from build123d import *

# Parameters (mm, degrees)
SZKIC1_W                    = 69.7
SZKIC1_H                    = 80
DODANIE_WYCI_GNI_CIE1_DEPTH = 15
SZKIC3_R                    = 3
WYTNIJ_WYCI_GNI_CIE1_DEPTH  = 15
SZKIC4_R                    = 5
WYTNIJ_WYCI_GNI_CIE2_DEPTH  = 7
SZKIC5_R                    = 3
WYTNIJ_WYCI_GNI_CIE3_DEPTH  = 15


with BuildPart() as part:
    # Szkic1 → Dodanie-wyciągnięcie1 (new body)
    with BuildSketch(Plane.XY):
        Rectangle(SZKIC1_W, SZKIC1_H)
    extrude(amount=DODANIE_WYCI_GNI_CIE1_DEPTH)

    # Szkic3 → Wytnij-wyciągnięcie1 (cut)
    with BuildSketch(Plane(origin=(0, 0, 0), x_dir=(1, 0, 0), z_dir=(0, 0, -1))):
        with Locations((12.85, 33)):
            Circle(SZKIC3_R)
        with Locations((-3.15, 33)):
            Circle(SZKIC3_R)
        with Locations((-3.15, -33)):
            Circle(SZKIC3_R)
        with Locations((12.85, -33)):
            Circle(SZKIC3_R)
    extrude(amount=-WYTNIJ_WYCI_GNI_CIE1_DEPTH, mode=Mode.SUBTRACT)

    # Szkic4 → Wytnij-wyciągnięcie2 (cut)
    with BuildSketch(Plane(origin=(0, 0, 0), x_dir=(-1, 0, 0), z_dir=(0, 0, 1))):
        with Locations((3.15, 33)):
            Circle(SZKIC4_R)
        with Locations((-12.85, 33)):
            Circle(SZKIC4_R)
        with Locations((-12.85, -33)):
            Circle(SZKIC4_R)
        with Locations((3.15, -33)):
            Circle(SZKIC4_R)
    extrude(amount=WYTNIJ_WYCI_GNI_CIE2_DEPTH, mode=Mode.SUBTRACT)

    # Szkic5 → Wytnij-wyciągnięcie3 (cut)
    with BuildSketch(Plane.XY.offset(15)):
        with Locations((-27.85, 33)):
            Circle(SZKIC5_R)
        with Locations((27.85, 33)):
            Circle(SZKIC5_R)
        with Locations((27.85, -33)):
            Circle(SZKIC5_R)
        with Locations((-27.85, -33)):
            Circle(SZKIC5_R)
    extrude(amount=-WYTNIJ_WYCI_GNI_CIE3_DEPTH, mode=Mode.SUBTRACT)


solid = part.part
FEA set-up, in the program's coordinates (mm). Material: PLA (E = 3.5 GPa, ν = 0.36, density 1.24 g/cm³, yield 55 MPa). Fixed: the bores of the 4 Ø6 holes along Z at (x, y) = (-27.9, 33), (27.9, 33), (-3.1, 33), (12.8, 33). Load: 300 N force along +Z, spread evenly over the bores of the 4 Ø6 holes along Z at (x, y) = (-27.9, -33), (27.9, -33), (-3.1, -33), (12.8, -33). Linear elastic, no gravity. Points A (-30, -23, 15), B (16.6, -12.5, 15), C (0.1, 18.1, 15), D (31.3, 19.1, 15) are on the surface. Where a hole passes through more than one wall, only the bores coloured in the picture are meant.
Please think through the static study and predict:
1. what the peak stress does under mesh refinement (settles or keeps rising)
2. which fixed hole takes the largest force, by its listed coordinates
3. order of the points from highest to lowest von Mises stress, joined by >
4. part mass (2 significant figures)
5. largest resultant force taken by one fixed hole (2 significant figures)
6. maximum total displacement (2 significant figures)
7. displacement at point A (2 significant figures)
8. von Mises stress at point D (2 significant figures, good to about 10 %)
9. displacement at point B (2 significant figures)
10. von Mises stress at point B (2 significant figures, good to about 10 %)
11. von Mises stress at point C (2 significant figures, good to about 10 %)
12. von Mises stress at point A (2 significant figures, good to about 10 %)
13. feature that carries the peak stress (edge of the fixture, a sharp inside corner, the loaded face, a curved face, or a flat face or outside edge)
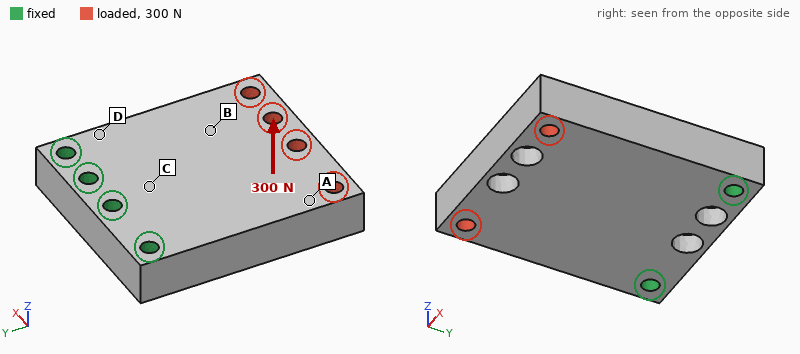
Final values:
keeps rising
(27.9, 33)
D > C > B > A
98 g
270 N
0.58 mm
0.38 mm
6.5 MPa
0.29 mm
2.5 MPa
5.2 MPa
1.3 MPa
edge of the fixture
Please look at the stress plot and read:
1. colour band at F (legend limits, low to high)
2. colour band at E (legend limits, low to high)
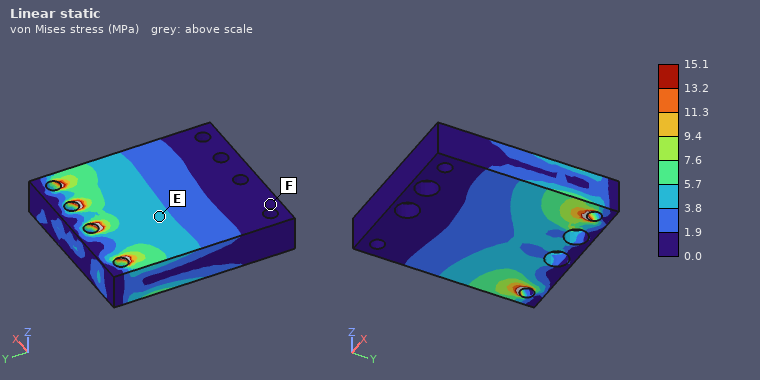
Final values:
0.0 to 1.9 MPa
3.8 to 5.7 MPa
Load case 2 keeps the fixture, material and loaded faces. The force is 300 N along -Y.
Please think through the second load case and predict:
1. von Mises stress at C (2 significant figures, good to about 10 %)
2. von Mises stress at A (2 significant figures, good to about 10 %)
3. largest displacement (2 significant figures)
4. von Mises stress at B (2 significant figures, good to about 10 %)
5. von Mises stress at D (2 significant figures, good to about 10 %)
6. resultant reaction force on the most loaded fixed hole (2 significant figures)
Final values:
0.40 MPa
0.44 MPa
14 µm
0.45 MPa
0.44 MPa
91 N
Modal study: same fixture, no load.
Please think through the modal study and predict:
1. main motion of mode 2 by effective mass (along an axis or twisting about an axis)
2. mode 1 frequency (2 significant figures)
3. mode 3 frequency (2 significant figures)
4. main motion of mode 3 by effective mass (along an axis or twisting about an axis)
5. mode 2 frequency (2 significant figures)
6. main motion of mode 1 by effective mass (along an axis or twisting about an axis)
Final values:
twisting about Y
720 Hz
2400 Hz
along X
1700 Hz
along Z
